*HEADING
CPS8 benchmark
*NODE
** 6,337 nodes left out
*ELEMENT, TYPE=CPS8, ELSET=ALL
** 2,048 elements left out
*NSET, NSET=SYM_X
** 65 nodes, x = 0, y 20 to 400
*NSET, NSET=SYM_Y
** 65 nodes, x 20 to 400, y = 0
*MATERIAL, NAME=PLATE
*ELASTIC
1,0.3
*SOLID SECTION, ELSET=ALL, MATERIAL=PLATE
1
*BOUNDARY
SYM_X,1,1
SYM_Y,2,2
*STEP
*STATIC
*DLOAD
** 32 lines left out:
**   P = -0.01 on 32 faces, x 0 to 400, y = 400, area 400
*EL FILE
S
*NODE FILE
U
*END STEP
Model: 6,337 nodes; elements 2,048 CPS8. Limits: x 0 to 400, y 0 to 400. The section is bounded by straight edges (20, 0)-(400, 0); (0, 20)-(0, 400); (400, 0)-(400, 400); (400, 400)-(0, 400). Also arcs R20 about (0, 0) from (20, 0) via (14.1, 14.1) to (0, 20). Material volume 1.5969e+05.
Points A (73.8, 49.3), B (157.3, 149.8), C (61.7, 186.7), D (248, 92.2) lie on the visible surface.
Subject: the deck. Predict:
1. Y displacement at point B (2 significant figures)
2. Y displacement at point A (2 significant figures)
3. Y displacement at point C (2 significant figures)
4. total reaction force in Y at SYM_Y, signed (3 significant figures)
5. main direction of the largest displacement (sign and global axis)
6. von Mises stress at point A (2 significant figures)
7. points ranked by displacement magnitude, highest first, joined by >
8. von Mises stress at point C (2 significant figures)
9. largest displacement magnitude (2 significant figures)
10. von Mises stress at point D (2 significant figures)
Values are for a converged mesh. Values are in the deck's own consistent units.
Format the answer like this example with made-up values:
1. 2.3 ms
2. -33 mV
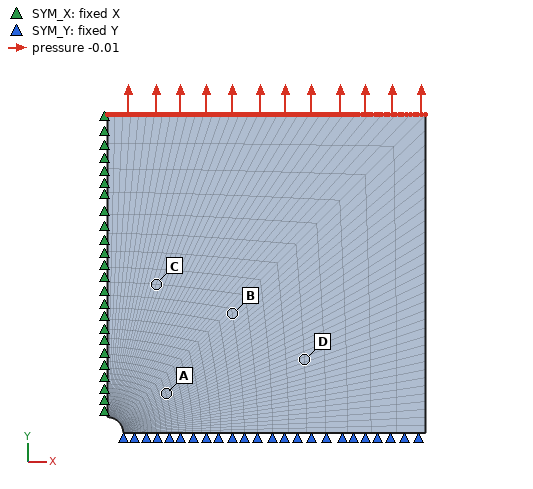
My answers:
1. 1.5
2. 0.52
3. 1.9
4. -4.00
5. +Y
6. 0.011
7. C > B > D > A
8. 0.0099
9. 4.2
10. 0.010
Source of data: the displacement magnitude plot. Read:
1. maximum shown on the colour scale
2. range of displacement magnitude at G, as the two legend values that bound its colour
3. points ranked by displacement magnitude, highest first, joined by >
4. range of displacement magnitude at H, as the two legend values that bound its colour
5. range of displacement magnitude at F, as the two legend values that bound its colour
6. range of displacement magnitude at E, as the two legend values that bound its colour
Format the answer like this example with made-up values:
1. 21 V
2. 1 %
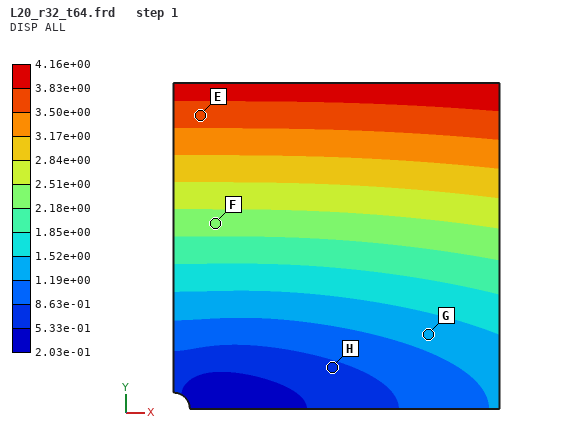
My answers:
1. 4.16e+00
2. 1.19e+00 to 1.52e+00
3. E > F > G > H
4. 5.33e-01 to 8.63e-01
5. 2.18e+00 to 2.51e+00
6. 3.50e+00 to 3.83e+00
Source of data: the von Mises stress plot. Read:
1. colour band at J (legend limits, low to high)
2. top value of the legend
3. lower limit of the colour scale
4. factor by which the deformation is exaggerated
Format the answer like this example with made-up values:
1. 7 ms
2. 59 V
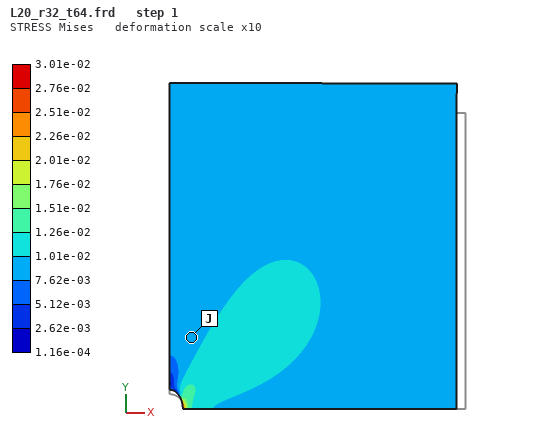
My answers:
1. 7.62e-03 to 1.01e-02
2. 3.01e-02
3. 1.16e-04
4. 10
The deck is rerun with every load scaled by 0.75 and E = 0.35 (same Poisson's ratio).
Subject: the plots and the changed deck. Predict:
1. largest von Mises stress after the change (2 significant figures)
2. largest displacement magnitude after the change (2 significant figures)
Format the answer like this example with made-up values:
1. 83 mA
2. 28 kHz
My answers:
1. 0.023
2. 8.9
